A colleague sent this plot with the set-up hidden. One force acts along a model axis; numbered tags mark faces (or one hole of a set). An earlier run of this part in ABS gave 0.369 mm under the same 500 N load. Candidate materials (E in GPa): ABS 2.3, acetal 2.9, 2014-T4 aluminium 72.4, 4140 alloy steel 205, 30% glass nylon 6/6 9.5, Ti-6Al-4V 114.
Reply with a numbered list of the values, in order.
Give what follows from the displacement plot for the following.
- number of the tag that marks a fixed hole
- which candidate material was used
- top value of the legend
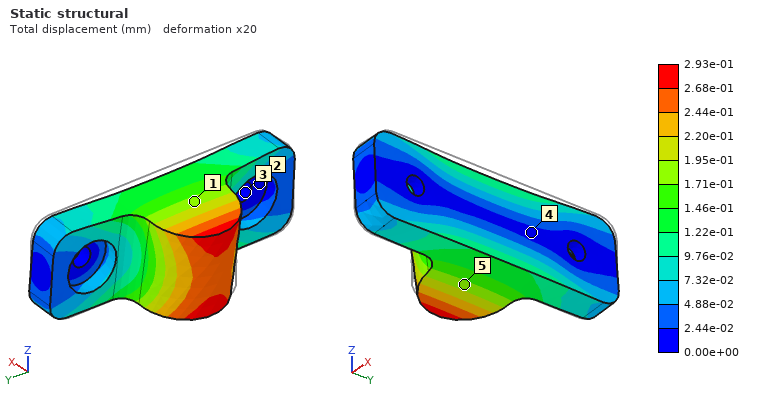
1. 3
2. acetal
3. 2.93e-01 mm
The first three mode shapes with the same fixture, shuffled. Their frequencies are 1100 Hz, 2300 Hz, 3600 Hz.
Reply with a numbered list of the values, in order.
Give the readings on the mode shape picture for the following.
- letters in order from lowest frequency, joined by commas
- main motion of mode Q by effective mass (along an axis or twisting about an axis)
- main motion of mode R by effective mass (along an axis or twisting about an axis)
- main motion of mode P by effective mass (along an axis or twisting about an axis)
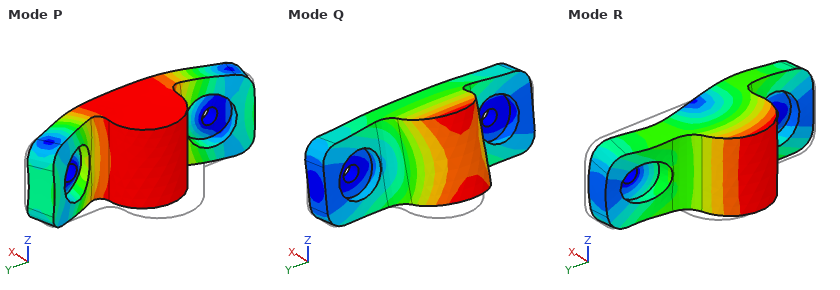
1. Q, P, R
2. along Z
3. along Y
4. along X
